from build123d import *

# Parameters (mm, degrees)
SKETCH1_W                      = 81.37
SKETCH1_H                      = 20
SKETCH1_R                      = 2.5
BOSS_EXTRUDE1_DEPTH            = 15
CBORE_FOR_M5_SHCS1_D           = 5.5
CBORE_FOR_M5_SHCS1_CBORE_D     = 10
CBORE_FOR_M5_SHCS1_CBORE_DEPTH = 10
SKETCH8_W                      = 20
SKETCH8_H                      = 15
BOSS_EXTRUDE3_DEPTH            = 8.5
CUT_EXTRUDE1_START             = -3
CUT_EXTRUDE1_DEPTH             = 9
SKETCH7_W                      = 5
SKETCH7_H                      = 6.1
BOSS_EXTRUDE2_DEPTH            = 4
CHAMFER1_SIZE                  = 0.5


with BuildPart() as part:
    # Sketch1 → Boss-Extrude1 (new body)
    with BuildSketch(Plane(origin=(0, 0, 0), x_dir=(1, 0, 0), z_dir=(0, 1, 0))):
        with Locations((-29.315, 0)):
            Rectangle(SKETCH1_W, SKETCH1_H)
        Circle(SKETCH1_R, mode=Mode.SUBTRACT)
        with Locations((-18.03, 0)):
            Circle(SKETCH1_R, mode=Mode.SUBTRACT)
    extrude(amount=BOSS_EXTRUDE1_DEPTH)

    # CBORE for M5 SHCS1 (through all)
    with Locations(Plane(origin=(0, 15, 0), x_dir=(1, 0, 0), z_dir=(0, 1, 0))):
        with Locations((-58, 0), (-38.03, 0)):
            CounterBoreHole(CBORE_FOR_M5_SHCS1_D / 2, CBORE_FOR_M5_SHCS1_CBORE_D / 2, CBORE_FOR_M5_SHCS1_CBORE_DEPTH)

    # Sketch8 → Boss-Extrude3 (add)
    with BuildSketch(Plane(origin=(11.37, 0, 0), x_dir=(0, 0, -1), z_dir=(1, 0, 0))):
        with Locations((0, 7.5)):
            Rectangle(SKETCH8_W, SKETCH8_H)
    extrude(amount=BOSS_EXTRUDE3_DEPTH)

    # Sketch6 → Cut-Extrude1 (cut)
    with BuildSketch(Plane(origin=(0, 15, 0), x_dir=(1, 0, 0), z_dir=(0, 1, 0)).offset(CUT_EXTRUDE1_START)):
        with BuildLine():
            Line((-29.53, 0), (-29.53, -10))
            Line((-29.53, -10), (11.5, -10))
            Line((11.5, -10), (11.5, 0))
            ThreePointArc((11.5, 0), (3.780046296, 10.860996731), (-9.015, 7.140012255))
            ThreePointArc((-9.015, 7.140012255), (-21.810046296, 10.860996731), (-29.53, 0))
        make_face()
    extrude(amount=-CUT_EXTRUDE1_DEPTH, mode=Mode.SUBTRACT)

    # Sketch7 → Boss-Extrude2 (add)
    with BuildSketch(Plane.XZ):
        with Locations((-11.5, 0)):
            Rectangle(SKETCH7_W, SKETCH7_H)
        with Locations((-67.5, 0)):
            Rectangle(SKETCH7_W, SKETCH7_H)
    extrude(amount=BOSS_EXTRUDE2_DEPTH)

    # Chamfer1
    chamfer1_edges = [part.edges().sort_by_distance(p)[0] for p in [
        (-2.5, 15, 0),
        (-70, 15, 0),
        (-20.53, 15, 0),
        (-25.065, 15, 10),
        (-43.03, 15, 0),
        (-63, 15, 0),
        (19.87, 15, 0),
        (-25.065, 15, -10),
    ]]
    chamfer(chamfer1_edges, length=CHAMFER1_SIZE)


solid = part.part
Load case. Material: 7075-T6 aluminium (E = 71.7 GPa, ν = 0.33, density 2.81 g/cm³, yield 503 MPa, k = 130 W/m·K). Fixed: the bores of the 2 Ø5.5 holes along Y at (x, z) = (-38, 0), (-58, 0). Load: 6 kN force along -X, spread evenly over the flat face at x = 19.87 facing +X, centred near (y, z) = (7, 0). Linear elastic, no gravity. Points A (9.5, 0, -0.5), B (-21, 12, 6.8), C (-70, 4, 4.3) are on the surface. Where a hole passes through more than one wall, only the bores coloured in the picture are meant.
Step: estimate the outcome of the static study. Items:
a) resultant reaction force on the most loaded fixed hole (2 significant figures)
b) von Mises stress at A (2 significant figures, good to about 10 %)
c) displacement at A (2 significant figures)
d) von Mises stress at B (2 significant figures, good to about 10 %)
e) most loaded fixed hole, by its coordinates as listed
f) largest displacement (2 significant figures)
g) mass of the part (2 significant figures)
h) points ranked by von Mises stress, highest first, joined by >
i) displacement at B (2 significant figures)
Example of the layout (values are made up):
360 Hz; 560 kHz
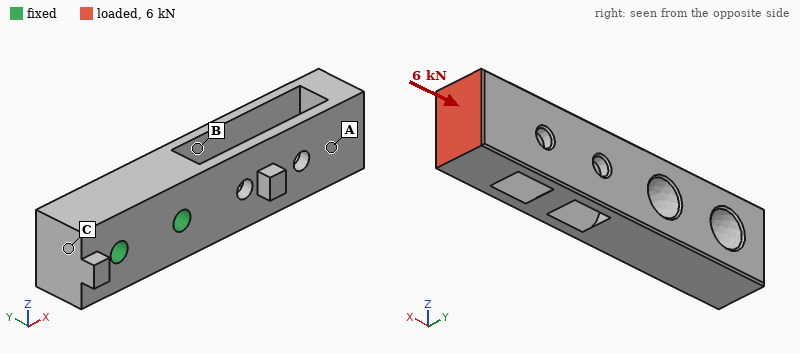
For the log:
4.2 kN; 36 MPa; 49 µm; 65 MPa; (-38, 0); 68 µm; 51 g; B > A > C; 29 µm
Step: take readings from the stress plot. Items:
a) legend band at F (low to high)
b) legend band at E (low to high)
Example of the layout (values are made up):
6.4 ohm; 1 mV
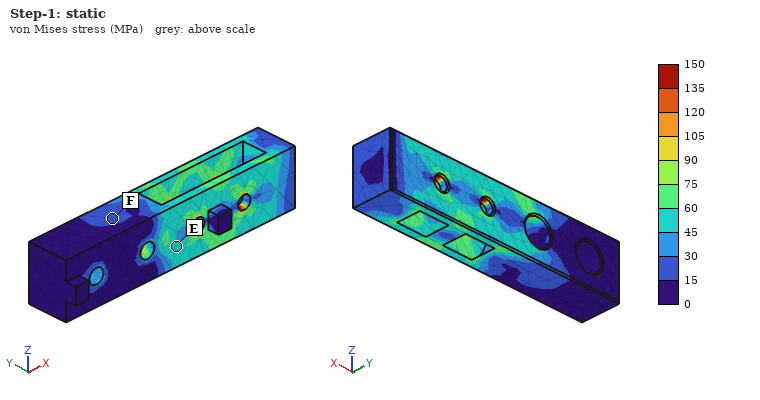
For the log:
15 to 30 MPa; 45 to 60 MPa
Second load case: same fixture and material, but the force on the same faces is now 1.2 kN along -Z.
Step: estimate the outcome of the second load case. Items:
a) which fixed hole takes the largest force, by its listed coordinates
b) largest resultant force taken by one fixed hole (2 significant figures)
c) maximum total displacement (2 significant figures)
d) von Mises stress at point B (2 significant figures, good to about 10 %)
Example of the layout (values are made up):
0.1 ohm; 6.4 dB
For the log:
(-38, 0); 3.6 kN; 0.34 mm; 91 MPa
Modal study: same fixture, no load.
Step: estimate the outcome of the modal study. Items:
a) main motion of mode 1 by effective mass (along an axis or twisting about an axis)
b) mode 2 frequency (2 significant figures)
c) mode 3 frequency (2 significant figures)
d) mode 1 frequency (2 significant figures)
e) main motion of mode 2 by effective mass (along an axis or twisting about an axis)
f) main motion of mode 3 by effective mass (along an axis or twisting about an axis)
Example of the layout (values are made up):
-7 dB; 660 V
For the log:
along Y; 3200 Hz; 5500 Hz; 1600 Hz; along Z; twisting about X
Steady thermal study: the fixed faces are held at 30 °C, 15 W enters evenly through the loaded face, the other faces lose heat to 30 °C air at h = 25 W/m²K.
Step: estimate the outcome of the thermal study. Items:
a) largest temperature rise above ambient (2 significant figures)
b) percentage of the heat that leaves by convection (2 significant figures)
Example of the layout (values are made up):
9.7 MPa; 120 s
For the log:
45 K; 22 %
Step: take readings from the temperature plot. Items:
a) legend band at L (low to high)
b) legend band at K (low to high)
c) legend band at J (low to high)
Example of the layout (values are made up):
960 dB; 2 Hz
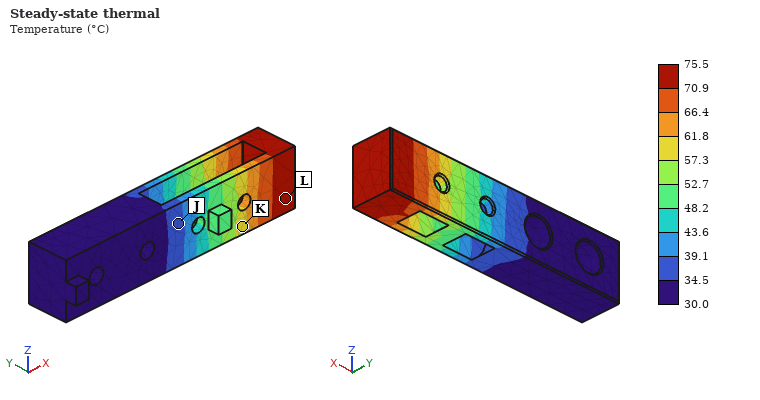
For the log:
70.9 to 75.5 °C; 57.3 to 61.8 °C; 34.5 to 39.1 °C
